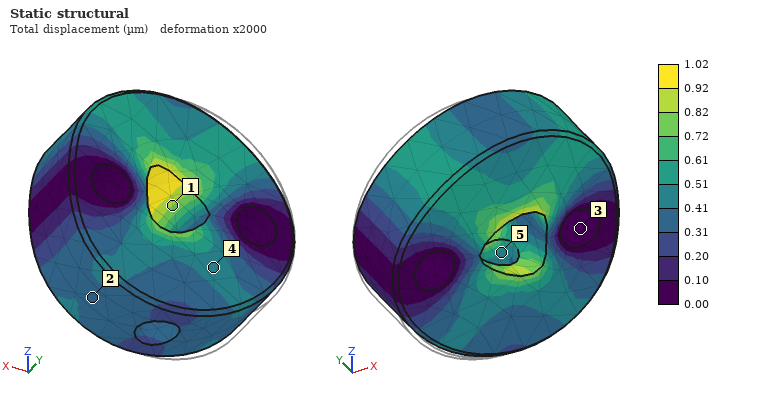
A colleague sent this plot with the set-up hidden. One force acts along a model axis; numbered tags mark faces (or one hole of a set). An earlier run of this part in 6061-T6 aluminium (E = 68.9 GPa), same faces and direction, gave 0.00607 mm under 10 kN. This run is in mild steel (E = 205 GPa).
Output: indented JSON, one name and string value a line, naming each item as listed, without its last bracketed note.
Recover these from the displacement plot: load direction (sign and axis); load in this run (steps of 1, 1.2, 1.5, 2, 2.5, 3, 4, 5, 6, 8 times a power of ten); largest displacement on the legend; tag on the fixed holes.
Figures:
{
  "load direction": "+X",
  "load in this run": "5 kN",
  "largest displacement on the legend": "1.02 µm",
  "tag on the fixed holes": "3"
}
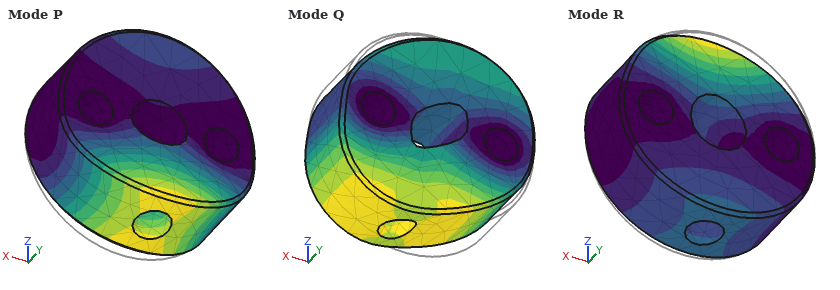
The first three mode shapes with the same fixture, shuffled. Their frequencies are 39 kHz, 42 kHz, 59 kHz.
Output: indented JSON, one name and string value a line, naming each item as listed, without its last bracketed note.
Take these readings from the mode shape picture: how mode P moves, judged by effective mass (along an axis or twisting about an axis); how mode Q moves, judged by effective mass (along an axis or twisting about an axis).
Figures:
{
  "how mode P moves, judged by effective mass": "along Y",
  "how mode Q moves, judged by effective mass": "twisting about Y"
}
